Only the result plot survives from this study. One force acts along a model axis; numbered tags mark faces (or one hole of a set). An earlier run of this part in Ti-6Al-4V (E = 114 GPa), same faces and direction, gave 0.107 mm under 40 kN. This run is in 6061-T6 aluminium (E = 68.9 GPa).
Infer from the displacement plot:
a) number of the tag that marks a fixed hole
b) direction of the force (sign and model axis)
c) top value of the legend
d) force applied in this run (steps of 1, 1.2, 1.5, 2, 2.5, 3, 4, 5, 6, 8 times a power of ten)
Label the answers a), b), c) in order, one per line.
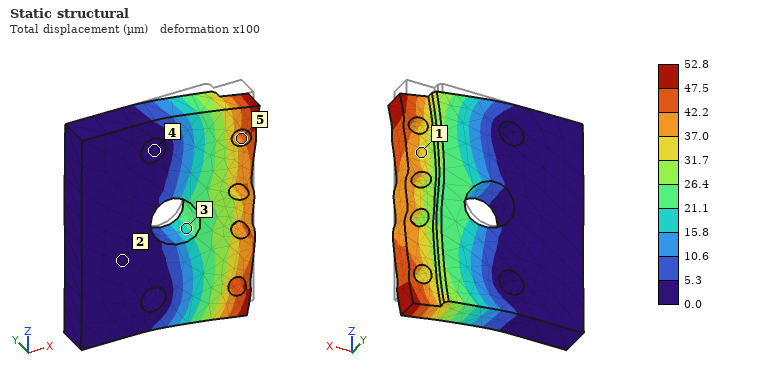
a) 4
b) -Z
c) 52.8 µm
d) 12 kN
